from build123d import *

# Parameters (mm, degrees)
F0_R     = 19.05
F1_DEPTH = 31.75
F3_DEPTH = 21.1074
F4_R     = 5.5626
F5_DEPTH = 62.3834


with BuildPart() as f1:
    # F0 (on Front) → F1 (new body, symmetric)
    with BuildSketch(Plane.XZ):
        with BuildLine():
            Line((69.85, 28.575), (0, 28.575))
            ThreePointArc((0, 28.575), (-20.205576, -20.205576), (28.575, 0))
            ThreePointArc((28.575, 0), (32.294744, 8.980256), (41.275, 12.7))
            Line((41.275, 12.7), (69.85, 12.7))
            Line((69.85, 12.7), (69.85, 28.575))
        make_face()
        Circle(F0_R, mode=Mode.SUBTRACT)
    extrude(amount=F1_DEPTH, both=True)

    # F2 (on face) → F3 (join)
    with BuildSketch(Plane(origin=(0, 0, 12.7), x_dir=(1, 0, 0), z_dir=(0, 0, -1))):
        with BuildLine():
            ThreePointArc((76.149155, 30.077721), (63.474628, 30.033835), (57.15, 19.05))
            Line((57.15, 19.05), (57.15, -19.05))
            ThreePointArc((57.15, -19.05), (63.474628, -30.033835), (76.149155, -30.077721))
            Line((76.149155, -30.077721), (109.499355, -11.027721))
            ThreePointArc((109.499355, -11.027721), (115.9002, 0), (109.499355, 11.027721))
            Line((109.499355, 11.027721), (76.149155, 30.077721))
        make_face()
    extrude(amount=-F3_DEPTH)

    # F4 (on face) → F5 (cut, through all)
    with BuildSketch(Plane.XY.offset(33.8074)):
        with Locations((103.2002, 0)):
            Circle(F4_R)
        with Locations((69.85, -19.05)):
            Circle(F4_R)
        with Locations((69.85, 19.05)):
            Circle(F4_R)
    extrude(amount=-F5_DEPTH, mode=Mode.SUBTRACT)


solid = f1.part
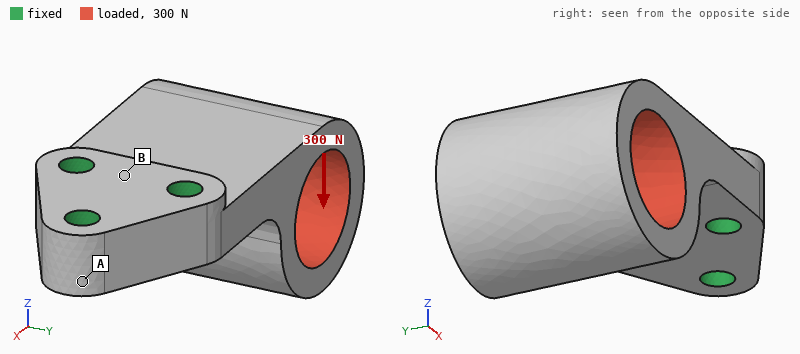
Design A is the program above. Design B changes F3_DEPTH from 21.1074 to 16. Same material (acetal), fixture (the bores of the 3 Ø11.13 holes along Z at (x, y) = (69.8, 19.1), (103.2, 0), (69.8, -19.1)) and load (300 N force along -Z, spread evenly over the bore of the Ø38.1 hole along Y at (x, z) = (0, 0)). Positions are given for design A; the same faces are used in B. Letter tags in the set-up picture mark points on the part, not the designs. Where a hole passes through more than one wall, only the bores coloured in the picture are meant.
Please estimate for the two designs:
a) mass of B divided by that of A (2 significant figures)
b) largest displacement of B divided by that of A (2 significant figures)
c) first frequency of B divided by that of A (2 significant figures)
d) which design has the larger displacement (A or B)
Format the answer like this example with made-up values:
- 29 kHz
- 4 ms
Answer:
- 0.94
- 1.1
- 0.94
- B
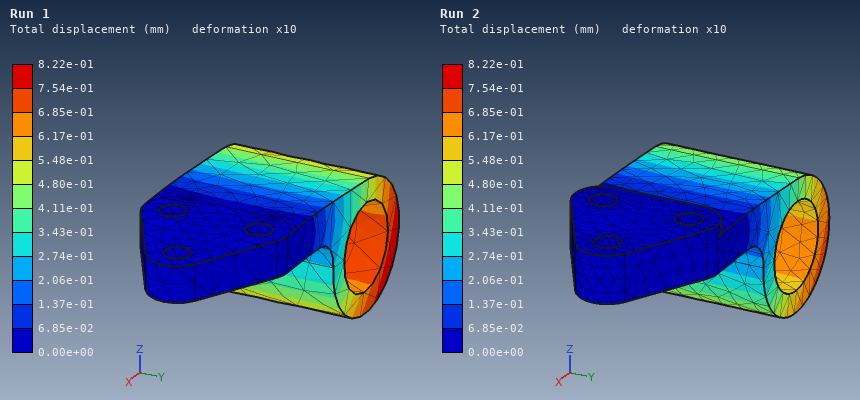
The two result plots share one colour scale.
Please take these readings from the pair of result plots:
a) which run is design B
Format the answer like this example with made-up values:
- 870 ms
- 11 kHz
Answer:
- Run 1
